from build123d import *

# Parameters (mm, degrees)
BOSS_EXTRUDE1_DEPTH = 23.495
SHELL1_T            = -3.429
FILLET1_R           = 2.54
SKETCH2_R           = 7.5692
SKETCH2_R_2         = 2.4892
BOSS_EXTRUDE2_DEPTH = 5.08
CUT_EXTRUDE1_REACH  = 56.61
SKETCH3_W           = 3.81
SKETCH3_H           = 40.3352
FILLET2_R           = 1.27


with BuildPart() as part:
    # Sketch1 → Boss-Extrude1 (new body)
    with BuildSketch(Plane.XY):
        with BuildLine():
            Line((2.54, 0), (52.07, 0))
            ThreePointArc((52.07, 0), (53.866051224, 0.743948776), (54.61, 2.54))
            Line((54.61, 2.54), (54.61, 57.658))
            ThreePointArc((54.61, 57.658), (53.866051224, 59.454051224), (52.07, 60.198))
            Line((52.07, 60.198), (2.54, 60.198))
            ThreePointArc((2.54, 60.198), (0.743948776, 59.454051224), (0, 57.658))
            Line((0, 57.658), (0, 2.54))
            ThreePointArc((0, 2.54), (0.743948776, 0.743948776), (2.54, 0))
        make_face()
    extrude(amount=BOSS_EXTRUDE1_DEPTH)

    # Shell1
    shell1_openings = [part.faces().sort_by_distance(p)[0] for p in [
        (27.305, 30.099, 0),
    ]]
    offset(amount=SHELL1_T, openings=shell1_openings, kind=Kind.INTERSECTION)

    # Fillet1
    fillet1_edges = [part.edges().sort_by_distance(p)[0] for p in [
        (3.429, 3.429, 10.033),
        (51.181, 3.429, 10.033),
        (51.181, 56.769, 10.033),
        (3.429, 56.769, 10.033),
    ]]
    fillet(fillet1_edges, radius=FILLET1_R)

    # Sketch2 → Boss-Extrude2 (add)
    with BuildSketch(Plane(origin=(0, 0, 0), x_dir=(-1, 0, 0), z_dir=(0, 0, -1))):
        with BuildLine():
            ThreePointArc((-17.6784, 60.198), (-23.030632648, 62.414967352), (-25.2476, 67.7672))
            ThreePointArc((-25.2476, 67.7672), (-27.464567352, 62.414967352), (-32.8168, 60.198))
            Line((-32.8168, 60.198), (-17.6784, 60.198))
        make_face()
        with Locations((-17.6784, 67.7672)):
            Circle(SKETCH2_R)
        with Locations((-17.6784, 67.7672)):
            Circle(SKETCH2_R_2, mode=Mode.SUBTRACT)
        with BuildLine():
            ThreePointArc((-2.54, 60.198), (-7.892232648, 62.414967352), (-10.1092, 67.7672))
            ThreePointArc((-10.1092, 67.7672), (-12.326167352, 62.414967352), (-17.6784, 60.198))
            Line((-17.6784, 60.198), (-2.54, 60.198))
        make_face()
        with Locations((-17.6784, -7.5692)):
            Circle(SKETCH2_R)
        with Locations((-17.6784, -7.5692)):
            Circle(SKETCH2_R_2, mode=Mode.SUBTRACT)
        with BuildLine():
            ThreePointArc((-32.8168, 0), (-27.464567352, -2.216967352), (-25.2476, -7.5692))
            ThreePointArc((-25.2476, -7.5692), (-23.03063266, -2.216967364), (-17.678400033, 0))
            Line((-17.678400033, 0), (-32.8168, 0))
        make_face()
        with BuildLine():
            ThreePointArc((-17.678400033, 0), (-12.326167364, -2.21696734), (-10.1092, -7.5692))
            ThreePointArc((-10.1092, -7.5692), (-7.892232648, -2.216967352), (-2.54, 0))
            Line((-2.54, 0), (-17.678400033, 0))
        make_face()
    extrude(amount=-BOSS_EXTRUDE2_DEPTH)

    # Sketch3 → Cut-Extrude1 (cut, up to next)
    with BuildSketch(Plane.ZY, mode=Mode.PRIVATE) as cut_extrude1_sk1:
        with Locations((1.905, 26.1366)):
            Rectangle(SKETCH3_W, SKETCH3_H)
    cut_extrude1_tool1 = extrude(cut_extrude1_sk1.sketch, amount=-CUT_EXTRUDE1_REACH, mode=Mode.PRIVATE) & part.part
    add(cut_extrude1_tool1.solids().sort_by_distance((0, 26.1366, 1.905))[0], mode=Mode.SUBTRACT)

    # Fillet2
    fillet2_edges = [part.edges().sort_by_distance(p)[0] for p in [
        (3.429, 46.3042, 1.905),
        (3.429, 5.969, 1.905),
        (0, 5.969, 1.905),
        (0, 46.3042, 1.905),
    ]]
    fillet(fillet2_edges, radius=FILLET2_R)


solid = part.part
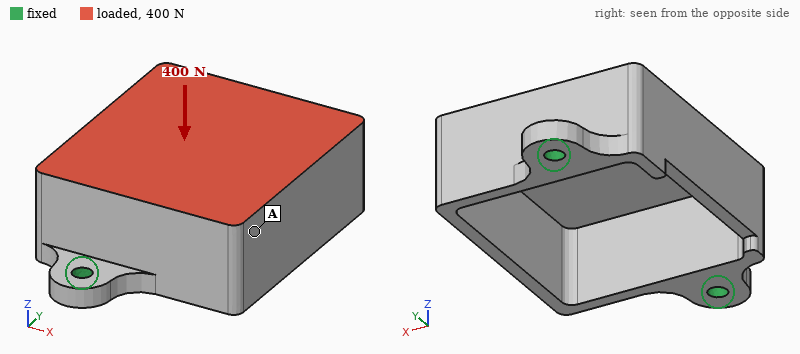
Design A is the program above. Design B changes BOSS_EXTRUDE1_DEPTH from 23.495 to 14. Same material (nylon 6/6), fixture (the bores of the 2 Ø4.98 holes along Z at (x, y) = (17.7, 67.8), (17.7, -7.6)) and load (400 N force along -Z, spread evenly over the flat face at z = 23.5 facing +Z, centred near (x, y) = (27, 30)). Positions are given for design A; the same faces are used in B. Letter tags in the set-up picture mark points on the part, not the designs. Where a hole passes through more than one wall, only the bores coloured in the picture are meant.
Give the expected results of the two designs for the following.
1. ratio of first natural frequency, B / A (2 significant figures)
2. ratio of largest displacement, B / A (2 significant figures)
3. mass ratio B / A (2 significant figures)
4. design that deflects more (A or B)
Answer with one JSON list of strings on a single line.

["1.3", "1.1", "0.75", "B"]
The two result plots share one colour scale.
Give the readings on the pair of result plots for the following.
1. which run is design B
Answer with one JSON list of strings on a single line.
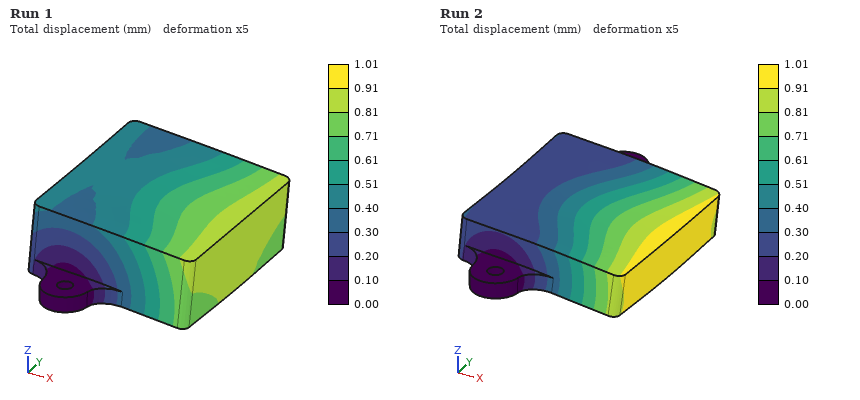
["Run 2"]
